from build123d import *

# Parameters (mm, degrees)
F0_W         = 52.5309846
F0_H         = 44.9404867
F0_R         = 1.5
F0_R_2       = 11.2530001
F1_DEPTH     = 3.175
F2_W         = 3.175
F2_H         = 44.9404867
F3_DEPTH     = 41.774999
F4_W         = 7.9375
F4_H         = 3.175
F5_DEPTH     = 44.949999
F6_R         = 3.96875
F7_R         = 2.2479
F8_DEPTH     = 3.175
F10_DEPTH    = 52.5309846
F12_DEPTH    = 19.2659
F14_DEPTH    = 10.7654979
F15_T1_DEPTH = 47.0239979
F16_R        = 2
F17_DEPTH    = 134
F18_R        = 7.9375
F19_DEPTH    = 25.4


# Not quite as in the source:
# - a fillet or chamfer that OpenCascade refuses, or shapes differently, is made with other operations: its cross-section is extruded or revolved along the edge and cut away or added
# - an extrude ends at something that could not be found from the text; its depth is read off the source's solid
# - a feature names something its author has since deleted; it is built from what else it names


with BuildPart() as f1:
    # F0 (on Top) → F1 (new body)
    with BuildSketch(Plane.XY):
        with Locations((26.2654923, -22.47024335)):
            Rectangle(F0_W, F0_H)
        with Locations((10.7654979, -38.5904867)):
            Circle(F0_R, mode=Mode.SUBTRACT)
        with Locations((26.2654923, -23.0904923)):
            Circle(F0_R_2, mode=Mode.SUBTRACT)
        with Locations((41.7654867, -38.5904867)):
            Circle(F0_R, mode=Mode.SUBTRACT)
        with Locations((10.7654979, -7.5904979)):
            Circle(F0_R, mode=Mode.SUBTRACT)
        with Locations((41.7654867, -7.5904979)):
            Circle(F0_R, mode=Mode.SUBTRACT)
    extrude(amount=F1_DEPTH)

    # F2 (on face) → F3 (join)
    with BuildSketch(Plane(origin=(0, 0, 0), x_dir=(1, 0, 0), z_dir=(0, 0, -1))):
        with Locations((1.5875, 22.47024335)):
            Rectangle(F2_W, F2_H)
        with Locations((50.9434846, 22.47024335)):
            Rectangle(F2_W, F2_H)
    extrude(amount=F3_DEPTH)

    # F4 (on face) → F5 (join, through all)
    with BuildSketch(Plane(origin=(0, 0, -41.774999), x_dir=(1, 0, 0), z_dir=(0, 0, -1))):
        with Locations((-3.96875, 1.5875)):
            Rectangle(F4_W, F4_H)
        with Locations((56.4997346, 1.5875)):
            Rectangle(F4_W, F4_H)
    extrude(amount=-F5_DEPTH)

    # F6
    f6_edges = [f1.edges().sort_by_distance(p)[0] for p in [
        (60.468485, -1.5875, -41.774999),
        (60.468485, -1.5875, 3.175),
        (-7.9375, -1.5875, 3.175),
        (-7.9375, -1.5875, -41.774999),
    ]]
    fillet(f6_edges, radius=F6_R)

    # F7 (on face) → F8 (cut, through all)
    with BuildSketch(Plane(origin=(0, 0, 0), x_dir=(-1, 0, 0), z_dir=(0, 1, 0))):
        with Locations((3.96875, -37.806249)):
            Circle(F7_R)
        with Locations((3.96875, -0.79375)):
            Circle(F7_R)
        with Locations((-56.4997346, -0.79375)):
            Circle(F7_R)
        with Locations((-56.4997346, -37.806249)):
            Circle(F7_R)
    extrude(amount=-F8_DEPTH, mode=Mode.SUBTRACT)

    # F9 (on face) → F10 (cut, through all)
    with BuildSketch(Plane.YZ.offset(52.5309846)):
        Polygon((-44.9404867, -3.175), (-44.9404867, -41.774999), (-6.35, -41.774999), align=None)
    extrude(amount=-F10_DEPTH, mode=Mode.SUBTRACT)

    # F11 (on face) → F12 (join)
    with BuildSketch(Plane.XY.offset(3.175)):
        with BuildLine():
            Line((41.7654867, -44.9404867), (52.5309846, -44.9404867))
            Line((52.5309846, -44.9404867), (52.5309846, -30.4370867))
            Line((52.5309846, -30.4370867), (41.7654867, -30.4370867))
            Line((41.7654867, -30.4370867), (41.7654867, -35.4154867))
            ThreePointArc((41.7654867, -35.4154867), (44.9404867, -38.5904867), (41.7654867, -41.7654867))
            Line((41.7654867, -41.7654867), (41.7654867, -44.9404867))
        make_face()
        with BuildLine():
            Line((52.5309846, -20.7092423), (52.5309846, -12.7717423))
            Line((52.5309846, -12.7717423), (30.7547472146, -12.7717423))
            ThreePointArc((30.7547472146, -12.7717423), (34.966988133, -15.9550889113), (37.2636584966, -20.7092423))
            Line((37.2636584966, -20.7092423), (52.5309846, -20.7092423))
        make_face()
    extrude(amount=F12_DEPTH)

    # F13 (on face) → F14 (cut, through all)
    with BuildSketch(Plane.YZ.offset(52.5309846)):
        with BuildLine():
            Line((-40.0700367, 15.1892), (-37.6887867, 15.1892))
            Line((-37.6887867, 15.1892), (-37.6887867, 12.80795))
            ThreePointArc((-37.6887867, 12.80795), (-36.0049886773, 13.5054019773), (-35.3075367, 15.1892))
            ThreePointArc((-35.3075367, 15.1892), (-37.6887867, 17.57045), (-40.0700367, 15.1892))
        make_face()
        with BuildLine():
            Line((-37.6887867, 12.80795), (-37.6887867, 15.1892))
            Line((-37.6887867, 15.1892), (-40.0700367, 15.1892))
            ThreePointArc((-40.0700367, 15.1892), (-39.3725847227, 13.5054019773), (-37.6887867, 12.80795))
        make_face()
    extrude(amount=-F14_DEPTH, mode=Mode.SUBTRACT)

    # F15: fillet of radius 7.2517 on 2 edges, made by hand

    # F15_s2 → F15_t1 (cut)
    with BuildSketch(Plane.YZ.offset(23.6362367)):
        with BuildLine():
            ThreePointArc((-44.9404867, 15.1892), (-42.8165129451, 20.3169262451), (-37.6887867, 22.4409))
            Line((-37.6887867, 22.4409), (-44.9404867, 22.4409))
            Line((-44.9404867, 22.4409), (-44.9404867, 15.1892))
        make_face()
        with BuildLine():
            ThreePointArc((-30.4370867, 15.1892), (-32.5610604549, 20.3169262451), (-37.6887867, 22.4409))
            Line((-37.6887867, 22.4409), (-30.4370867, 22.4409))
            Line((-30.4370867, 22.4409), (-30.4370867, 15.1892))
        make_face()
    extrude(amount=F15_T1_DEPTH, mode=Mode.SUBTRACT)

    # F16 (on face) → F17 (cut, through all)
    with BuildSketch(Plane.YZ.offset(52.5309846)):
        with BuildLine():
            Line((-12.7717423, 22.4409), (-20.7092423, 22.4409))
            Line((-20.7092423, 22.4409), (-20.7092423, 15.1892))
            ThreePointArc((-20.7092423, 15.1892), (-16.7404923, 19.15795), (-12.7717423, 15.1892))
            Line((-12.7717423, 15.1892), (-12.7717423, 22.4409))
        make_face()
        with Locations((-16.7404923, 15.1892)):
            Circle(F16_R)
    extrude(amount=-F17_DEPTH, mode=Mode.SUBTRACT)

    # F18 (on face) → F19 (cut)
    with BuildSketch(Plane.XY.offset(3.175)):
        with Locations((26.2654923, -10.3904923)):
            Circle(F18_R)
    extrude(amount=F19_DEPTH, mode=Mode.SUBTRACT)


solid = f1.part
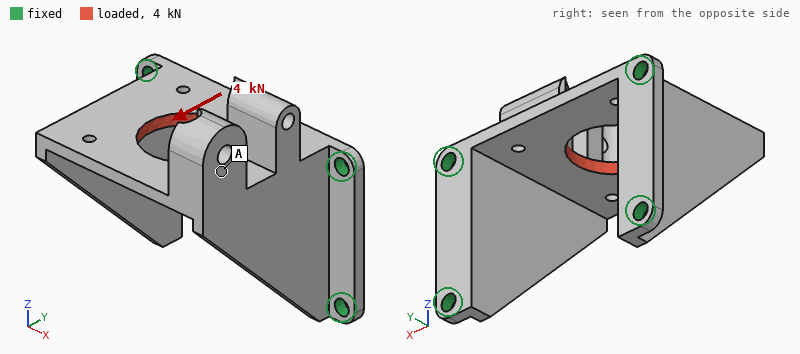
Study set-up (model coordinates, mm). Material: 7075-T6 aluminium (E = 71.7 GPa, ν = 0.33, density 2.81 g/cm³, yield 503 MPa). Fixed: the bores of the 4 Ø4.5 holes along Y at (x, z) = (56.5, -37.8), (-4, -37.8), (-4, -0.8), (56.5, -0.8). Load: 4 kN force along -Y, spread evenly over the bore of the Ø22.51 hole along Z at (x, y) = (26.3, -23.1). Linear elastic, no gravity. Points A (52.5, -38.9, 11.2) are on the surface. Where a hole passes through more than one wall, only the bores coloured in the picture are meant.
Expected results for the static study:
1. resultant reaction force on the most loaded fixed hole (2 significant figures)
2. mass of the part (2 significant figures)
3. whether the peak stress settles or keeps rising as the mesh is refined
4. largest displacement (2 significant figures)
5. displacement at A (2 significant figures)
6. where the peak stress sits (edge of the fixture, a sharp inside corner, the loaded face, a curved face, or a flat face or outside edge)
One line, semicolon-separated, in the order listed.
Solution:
2.3 kN; 55 g; keeps rising; 77 µm; 60 µm; edge of the fixture
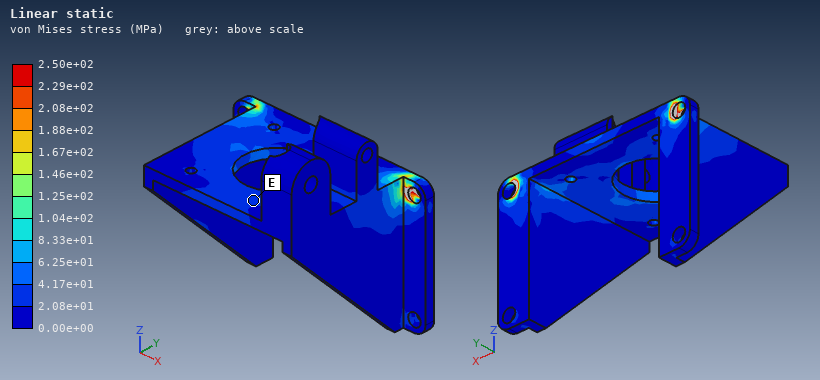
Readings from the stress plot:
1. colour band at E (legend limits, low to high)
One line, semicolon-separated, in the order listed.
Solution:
2.08e+01 to 4.17e+01 MPa
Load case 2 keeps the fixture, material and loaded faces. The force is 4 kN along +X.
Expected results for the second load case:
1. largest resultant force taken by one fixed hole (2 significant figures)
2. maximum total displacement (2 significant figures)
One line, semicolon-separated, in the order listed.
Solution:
2.6 kN; 93 µm
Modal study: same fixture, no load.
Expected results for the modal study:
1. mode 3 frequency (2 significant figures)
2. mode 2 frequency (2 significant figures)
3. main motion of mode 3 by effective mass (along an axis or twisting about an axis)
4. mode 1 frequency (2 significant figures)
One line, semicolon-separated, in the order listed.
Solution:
5800 Hz; 4800 Hz; along X; 3000 Hz
